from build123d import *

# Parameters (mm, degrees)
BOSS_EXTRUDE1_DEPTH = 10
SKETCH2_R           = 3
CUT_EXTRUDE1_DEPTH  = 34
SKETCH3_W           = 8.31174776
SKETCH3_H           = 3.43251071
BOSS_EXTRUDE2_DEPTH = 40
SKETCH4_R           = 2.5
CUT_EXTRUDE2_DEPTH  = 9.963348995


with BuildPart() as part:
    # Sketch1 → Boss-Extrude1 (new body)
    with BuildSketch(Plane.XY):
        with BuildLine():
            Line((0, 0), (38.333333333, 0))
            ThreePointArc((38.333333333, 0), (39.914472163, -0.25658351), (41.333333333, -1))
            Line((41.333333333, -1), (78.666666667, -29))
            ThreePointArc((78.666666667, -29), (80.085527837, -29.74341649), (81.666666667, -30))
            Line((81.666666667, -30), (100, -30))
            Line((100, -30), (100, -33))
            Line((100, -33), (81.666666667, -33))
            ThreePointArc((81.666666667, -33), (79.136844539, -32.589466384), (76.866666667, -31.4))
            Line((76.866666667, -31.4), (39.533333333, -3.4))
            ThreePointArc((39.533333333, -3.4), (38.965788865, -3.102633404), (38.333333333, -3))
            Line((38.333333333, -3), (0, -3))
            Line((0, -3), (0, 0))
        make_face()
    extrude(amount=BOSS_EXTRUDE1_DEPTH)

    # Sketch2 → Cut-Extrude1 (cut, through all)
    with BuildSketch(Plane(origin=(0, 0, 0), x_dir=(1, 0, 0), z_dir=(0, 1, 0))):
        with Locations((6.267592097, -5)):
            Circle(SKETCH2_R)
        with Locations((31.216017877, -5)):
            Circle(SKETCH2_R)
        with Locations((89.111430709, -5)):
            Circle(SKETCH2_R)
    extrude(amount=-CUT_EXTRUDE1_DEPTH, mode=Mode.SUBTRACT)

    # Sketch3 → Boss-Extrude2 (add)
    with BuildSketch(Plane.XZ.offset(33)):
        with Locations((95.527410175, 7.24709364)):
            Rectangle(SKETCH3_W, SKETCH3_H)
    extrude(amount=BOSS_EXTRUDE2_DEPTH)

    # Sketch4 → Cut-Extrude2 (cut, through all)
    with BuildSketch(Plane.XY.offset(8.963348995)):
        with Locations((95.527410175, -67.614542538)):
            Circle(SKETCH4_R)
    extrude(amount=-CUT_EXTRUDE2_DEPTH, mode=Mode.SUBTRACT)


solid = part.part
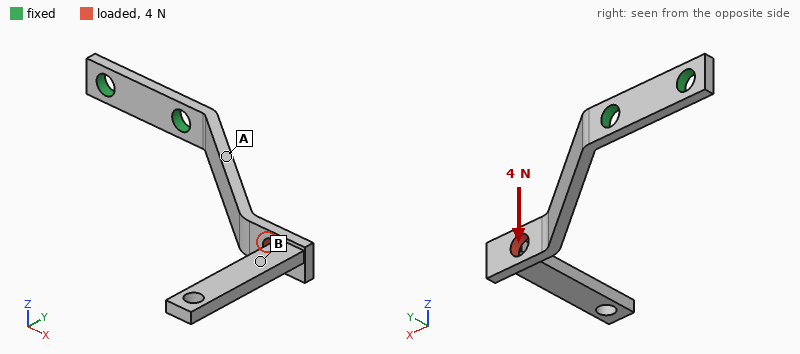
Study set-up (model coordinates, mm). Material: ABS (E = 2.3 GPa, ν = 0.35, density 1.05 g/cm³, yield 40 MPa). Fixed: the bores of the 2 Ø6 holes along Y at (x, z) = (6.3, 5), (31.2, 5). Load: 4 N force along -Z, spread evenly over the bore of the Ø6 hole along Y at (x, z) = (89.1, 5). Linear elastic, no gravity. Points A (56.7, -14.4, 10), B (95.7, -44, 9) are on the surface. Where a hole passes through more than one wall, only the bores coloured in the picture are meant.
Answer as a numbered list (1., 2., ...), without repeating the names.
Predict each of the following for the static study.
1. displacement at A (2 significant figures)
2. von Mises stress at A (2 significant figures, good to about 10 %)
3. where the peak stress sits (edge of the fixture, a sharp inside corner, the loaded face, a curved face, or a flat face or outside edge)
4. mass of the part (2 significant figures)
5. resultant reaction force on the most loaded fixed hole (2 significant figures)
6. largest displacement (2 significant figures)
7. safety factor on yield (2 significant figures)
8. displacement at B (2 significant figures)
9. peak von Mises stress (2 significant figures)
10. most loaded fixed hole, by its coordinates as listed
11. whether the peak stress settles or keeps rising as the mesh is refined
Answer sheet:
1. 0.25 mm
2. 3.0 MPa
3. a curved face
4. 4.3 g
5. 4.7 N
6. 1.2 mm
7. 3.7
8. 1.1 mm
9. 11 MPa
10. (31.2, 5)
11. settles
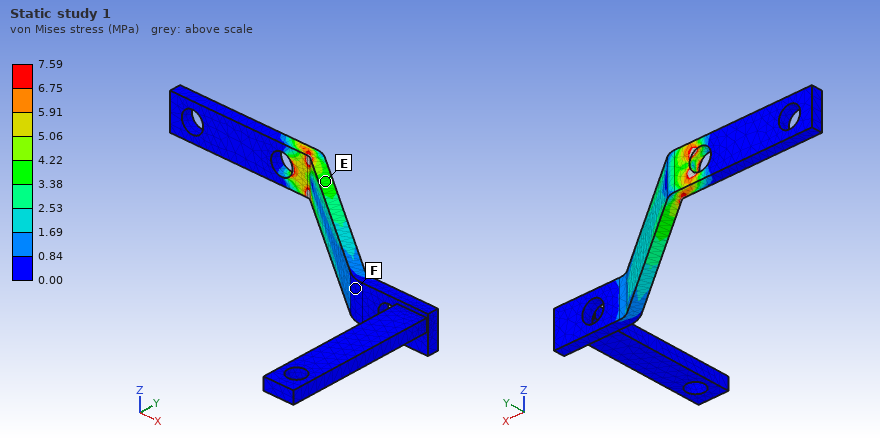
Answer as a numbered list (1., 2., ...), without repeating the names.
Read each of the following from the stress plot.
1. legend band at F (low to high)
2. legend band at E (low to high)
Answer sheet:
1. 0.00 to 0.84 MPa
2. 3.38 to 4.22 MPa
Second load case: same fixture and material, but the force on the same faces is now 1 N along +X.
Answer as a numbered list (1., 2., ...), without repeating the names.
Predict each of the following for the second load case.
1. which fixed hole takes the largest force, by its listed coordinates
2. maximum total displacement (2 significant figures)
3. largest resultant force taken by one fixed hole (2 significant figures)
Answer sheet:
1. (31.2, 5)
2. 1.4 mm
3. 0.99 N
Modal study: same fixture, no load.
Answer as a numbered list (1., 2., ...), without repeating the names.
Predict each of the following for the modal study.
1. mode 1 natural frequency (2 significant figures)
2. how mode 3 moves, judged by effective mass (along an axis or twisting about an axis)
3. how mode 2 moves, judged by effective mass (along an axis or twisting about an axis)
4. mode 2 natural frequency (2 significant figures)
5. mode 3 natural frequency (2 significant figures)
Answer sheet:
1. 68 Hz
2. along Y
3. along Z
4. 160 Hz
5. 350 Hz
